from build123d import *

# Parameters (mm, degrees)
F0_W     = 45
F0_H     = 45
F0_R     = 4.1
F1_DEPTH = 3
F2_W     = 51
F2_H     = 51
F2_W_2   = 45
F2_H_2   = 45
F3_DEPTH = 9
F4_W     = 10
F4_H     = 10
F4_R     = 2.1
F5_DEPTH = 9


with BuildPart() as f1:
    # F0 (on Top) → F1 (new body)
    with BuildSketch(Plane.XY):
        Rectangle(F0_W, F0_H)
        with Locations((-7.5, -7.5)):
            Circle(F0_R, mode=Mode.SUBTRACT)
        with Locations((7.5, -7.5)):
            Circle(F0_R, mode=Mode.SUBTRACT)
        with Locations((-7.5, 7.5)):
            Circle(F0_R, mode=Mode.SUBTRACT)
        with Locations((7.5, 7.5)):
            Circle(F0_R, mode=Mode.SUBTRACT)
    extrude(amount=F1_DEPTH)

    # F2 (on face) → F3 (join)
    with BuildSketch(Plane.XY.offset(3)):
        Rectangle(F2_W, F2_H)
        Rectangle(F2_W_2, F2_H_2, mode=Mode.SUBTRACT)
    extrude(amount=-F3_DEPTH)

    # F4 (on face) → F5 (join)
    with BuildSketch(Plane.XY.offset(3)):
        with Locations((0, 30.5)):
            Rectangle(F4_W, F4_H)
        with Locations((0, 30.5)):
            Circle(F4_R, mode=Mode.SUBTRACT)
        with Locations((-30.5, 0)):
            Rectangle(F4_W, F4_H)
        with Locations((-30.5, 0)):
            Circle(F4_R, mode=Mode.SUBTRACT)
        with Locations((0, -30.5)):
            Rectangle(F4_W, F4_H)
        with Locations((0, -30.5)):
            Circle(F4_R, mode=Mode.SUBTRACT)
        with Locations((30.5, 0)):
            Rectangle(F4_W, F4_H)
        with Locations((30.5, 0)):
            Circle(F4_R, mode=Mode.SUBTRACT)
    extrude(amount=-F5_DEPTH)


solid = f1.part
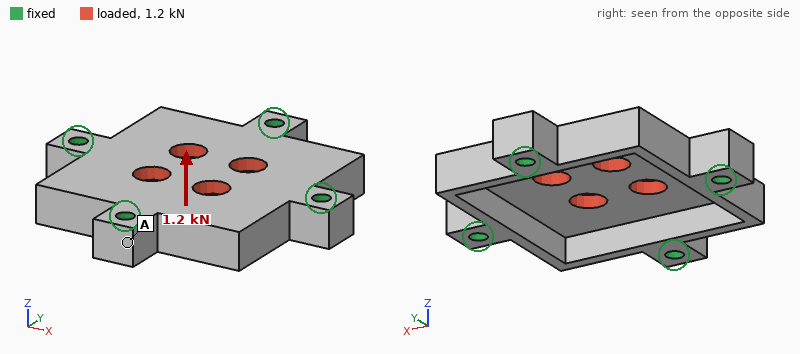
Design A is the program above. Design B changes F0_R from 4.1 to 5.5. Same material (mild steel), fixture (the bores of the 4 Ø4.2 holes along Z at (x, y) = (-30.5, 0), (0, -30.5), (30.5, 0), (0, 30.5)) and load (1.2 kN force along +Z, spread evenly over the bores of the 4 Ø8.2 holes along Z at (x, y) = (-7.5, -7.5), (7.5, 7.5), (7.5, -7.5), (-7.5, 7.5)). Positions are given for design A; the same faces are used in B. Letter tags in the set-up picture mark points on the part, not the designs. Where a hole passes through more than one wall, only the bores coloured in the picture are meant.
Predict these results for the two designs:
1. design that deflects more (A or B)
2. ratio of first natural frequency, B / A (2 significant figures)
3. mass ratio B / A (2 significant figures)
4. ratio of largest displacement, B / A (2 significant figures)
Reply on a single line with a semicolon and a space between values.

B; 1.1; 0.96; 1.2
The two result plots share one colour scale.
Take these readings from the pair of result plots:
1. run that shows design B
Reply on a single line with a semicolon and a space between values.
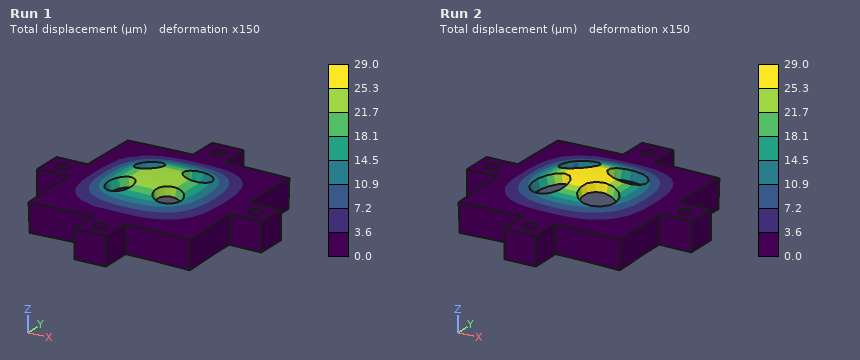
Run 2
